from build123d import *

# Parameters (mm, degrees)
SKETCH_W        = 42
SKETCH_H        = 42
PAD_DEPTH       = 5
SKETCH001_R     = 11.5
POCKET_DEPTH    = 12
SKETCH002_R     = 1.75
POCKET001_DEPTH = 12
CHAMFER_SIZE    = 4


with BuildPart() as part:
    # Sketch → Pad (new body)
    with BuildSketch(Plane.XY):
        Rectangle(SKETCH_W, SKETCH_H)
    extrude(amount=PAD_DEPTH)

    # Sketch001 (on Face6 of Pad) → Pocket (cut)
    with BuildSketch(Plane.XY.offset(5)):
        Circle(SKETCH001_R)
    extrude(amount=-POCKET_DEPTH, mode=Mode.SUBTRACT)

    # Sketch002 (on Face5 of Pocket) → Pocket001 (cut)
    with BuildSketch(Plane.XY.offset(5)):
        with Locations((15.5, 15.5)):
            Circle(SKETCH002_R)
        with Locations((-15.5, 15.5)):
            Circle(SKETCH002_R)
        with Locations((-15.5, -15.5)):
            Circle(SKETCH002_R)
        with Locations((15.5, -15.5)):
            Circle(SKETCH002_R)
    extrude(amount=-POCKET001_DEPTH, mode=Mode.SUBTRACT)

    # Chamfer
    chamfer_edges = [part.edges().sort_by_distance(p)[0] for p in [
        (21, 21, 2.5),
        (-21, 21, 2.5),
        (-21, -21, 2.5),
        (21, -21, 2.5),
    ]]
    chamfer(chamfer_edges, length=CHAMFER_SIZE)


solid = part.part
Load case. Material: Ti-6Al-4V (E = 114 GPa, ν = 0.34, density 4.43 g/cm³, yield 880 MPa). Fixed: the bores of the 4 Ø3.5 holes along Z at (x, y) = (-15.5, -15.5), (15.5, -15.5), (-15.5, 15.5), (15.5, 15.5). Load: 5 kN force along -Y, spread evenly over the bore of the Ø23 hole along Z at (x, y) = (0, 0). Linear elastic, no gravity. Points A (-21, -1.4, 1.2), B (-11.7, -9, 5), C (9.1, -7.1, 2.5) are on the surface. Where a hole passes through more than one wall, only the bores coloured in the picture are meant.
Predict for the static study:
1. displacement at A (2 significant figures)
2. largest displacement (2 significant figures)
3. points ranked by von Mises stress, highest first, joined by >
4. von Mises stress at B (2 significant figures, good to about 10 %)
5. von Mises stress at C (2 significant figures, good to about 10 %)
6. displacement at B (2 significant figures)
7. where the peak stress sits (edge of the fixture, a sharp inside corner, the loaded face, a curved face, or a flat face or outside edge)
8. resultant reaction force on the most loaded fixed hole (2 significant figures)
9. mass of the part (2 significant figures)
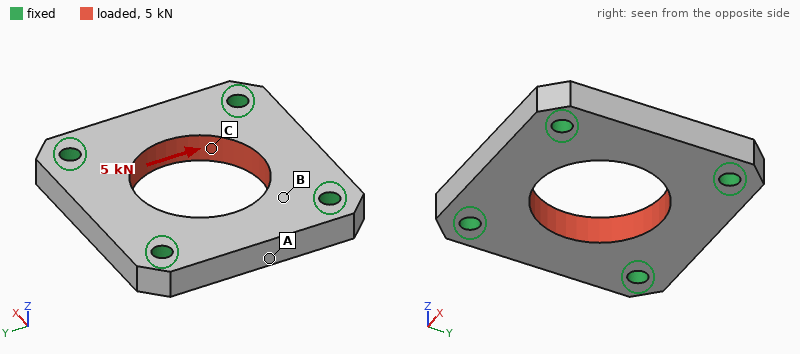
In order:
1.3 µm
5.8 µm
C > B > A
22 MPa
36 MPa
2.1 µm
edge of the fixture
1.3 kN
28 g
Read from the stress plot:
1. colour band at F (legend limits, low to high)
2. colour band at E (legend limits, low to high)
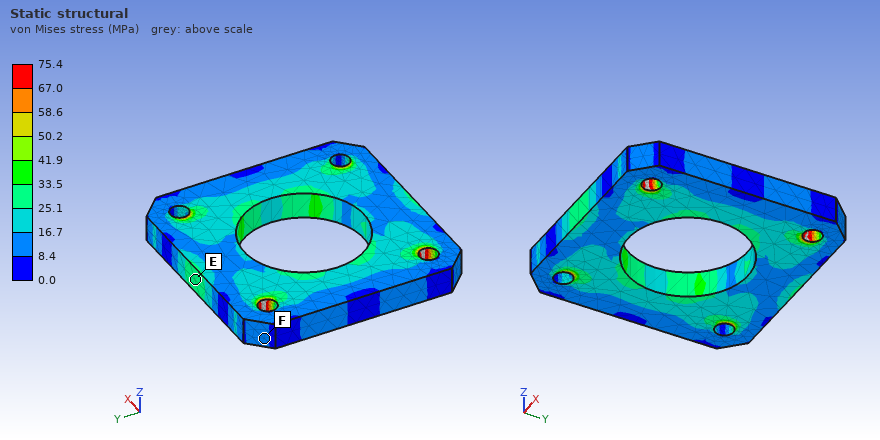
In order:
8.4 to 16.7 MPa
25.1 to 33.5 MPa
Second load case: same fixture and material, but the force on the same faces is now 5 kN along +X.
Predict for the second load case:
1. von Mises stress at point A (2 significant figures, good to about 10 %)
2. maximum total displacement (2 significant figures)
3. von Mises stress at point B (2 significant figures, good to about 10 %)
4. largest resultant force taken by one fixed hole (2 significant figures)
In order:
29 MPa
5.8 µm
19 MPa
1.3 kN
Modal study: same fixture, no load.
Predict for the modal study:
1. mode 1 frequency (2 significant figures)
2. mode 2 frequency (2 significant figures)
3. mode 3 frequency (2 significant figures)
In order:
24 kHz
25 kHz
26 kHz
